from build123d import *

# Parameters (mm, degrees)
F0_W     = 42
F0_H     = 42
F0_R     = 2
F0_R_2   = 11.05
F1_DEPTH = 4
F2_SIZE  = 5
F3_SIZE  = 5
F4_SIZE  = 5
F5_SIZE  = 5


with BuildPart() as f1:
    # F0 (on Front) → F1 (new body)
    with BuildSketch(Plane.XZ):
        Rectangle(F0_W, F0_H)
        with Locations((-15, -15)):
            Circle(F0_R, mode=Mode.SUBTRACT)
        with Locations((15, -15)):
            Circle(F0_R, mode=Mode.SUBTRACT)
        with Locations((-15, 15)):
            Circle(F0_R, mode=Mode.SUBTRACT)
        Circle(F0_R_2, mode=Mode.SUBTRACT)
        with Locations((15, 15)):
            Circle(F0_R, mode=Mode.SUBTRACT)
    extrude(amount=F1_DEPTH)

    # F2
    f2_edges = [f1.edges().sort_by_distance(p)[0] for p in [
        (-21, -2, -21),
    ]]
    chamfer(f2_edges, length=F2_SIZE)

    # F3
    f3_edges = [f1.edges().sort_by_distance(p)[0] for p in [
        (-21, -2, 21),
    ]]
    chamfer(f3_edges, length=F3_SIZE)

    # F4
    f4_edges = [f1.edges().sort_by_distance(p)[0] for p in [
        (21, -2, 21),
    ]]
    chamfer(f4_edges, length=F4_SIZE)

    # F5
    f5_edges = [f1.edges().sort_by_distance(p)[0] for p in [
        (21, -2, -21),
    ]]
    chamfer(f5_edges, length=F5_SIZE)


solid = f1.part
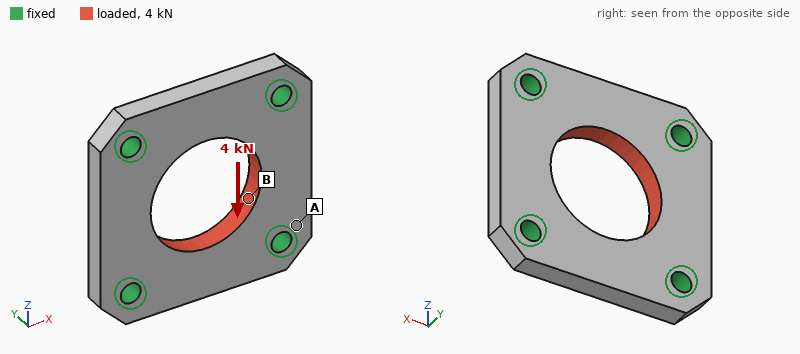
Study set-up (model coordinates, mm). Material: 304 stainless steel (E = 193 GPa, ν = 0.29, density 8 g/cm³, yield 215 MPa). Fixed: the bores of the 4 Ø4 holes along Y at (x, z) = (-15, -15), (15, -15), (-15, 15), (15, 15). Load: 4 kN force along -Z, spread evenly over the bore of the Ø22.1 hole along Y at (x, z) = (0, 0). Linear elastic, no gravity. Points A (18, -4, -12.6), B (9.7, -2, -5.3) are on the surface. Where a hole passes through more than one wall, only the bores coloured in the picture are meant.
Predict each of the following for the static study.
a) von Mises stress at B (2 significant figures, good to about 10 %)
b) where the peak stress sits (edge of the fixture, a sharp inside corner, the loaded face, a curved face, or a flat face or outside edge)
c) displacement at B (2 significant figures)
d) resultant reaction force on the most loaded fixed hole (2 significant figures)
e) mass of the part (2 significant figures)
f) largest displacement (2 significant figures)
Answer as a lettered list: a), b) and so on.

a) 30 MPa
b) edge of the fixture
c) 1.4 µm
d) 1.0 kN
e) 41 g
f) 2.9 µm
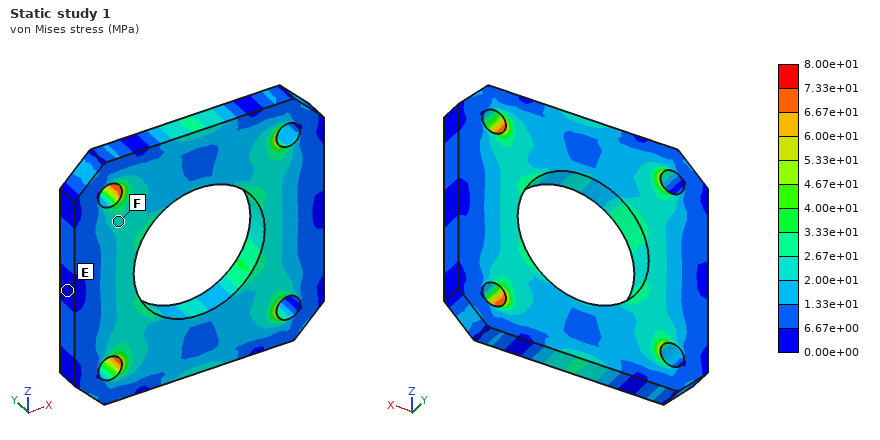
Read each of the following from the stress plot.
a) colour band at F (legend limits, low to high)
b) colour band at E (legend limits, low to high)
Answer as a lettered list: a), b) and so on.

a) 2.00e+01 to 2.67e+01 MPa
b) 0.00e+00 to 6.67e+00 MPa
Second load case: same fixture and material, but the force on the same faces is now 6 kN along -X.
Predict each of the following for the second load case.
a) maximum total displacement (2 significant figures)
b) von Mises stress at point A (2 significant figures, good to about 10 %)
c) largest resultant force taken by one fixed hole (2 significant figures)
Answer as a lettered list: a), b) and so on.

a) 4.4 µm
b) 25 MPa
c) 1.5 kN
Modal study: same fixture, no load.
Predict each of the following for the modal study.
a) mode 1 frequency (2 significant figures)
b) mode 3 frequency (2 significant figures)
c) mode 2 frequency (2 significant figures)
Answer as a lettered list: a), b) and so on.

a) 23 kHz
b) 23 kHz
c) 23 kHz
